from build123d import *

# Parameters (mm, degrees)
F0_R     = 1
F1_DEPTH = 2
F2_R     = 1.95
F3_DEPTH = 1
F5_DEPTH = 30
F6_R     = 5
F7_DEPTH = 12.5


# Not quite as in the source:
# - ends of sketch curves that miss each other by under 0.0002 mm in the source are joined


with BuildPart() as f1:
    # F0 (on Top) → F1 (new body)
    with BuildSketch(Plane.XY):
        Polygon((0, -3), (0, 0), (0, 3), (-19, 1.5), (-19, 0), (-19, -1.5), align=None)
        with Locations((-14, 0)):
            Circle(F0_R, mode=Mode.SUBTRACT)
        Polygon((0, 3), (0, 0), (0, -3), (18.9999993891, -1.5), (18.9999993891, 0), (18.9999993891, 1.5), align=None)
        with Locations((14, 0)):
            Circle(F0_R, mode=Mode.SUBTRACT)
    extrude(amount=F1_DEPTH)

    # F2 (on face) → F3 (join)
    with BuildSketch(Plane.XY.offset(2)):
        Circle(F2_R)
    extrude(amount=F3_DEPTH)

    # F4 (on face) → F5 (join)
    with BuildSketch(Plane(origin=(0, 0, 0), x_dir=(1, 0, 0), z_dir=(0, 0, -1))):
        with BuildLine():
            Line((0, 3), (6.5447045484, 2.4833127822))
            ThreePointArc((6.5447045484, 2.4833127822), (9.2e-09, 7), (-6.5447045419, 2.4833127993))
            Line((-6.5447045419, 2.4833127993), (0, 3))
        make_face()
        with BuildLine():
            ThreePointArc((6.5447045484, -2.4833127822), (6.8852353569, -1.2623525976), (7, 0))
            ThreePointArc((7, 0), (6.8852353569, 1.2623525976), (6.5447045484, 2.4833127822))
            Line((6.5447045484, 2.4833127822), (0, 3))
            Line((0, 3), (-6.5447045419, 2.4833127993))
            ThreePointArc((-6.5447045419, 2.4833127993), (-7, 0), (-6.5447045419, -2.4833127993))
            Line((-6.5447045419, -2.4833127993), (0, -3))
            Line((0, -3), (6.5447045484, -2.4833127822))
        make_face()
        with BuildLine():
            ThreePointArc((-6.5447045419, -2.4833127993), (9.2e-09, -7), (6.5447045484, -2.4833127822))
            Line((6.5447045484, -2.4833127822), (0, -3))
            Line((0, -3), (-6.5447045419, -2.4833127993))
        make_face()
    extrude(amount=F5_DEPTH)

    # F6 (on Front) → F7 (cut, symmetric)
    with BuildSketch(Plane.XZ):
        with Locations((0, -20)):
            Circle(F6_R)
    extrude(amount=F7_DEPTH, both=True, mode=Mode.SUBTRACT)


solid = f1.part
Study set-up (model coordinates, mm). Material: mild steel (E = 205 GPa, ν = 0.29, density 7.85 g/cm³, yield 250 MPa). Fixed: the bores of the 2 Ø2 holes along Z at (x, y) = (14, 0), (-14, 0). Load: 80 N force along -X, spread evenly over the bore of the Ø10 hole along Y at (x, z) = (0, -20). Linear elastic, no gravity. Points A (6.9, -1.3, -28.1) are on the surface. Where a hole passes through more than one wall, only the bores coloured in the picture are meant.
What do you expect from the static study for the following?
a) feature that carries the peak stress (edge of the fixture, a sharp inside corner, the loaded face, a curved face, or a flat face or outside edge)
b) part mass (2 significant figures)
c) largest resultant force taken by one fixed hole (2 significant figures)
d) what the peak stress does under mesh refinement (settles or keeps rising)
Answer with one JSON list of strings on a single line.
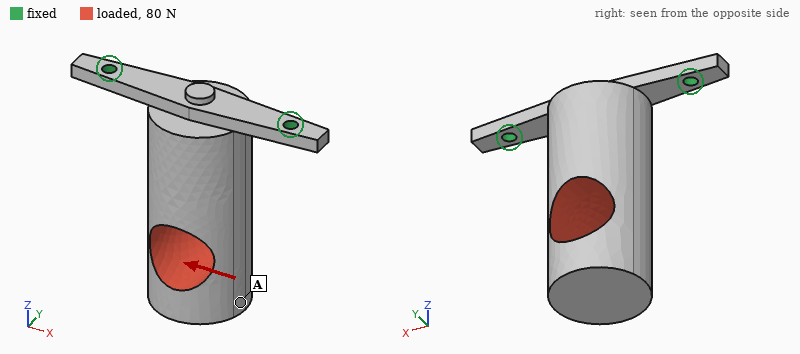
["edge of the fixture", "31 g", "90 N", "keeps rising"]
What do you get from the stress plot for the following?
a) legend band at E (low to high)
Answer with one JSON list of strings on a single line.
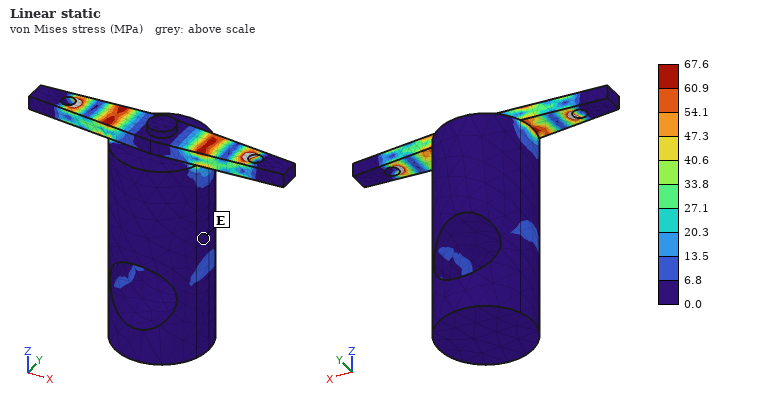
["0.0 to 6.8 MPa"]
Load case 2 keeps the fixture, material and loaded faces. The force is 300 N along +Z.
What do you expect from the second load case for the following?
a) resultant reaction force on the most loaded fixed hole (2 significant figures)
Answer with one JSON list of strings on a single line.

["170 N"]
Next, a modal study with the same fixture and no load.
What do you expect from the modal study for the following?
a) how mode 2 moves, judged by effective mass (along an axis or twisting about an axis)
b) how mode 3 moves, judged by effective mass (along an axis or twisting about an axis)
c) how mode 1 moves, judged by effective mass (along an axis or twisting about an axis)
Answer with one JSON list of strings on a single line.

["along X", "along Z", "along Y"]
